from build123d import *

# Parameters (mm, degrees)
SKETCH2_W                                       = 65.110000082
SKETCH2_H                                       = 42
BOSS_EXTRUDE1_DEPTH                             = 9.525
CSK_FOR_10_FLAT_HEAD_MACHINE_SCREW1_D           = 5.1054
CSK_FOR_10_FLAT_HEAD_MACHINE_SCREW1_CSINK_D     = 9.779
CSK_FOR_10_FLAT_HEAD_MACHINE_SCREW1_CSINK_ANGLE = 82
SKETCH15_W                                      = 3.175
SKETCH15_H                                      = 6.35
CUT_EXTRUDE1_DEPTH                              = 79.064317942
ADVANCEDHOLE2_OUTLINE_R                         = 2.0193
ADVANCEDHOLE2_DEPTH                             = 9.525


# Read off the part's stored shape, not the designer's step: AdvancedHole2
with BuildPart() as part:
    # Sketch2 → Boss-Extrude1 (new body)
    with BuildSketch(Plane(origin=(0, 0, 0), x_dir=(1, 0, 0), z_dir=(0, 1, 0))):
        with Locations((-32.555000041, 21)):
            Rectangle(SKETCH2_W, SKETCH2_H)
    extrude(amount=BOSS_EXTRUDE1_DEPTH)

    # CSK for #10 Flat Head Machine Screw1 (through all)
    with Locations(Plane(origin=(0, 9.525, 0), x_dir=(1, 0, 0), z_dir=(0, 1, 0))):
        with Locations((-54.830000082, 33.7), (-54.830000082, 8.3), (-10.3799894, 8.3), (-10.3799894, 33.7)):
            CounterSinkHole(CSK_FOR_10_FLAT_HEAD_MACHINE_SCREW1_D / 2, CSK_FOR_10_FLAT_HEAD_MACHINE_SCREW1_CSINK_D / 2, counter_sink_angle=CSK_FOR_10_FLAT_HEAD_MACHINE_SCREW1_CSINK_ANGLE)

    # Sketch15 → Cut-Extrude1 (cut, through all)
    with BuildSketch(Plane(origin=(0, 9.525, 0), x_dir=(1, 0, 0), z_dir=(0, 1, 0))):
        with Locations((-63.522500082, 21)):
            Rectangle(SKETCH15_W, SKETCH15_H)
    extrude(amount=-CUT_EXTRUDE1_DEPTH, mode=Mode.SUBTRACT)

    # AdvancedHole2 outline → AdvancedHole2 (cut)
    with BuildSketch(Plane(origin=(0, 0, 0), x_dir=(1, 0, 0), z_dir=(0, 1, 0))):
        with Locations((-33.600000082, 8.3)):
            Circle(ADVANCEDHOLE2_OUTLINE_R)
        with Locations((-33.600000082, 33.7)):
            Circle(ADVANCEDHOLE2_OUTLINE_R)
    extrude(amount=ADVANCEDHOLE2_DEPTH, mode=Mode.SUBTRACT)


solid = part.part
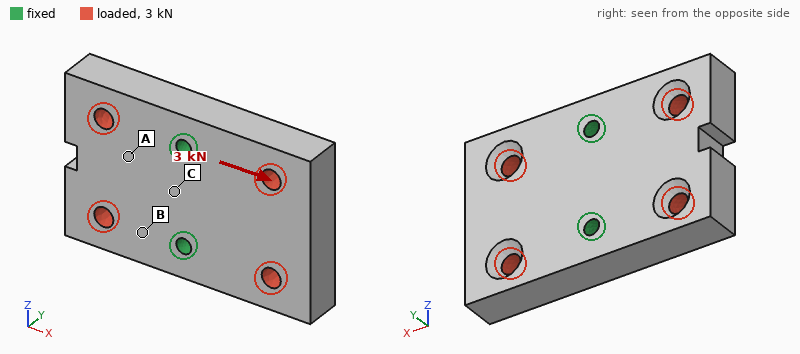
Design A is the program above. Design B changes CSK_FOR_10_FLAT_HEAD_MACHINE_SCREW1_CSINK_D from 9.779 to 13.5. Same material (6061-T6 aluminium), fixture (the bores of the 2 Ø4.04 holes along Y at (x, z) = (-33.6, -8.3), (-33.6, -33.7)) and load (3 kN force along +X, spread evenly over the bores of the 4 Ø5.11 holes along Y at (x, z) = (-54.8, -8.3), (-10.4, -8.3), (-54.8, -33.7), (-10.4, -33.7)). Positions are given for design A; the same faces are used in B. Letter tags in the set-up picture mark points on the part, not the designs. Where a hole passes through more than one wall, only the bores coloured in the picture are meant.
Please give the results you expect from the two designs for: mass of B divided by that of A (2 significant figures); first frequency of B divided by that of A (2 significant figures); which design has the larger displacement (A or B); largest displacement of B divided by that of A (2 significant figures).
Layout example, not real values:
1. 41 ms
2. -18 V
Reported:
1. 0.97
2. 1.0
3. B
4. 1.7
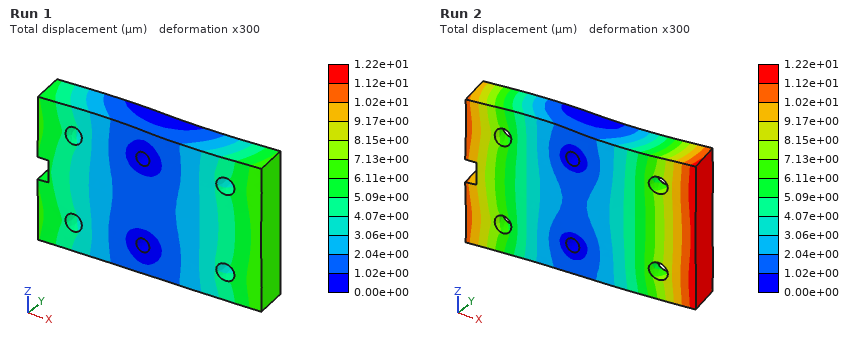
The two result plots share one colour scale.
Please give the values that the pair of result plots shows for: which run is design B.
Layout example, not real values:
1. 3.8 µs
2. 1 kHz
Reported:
1. Run 2
